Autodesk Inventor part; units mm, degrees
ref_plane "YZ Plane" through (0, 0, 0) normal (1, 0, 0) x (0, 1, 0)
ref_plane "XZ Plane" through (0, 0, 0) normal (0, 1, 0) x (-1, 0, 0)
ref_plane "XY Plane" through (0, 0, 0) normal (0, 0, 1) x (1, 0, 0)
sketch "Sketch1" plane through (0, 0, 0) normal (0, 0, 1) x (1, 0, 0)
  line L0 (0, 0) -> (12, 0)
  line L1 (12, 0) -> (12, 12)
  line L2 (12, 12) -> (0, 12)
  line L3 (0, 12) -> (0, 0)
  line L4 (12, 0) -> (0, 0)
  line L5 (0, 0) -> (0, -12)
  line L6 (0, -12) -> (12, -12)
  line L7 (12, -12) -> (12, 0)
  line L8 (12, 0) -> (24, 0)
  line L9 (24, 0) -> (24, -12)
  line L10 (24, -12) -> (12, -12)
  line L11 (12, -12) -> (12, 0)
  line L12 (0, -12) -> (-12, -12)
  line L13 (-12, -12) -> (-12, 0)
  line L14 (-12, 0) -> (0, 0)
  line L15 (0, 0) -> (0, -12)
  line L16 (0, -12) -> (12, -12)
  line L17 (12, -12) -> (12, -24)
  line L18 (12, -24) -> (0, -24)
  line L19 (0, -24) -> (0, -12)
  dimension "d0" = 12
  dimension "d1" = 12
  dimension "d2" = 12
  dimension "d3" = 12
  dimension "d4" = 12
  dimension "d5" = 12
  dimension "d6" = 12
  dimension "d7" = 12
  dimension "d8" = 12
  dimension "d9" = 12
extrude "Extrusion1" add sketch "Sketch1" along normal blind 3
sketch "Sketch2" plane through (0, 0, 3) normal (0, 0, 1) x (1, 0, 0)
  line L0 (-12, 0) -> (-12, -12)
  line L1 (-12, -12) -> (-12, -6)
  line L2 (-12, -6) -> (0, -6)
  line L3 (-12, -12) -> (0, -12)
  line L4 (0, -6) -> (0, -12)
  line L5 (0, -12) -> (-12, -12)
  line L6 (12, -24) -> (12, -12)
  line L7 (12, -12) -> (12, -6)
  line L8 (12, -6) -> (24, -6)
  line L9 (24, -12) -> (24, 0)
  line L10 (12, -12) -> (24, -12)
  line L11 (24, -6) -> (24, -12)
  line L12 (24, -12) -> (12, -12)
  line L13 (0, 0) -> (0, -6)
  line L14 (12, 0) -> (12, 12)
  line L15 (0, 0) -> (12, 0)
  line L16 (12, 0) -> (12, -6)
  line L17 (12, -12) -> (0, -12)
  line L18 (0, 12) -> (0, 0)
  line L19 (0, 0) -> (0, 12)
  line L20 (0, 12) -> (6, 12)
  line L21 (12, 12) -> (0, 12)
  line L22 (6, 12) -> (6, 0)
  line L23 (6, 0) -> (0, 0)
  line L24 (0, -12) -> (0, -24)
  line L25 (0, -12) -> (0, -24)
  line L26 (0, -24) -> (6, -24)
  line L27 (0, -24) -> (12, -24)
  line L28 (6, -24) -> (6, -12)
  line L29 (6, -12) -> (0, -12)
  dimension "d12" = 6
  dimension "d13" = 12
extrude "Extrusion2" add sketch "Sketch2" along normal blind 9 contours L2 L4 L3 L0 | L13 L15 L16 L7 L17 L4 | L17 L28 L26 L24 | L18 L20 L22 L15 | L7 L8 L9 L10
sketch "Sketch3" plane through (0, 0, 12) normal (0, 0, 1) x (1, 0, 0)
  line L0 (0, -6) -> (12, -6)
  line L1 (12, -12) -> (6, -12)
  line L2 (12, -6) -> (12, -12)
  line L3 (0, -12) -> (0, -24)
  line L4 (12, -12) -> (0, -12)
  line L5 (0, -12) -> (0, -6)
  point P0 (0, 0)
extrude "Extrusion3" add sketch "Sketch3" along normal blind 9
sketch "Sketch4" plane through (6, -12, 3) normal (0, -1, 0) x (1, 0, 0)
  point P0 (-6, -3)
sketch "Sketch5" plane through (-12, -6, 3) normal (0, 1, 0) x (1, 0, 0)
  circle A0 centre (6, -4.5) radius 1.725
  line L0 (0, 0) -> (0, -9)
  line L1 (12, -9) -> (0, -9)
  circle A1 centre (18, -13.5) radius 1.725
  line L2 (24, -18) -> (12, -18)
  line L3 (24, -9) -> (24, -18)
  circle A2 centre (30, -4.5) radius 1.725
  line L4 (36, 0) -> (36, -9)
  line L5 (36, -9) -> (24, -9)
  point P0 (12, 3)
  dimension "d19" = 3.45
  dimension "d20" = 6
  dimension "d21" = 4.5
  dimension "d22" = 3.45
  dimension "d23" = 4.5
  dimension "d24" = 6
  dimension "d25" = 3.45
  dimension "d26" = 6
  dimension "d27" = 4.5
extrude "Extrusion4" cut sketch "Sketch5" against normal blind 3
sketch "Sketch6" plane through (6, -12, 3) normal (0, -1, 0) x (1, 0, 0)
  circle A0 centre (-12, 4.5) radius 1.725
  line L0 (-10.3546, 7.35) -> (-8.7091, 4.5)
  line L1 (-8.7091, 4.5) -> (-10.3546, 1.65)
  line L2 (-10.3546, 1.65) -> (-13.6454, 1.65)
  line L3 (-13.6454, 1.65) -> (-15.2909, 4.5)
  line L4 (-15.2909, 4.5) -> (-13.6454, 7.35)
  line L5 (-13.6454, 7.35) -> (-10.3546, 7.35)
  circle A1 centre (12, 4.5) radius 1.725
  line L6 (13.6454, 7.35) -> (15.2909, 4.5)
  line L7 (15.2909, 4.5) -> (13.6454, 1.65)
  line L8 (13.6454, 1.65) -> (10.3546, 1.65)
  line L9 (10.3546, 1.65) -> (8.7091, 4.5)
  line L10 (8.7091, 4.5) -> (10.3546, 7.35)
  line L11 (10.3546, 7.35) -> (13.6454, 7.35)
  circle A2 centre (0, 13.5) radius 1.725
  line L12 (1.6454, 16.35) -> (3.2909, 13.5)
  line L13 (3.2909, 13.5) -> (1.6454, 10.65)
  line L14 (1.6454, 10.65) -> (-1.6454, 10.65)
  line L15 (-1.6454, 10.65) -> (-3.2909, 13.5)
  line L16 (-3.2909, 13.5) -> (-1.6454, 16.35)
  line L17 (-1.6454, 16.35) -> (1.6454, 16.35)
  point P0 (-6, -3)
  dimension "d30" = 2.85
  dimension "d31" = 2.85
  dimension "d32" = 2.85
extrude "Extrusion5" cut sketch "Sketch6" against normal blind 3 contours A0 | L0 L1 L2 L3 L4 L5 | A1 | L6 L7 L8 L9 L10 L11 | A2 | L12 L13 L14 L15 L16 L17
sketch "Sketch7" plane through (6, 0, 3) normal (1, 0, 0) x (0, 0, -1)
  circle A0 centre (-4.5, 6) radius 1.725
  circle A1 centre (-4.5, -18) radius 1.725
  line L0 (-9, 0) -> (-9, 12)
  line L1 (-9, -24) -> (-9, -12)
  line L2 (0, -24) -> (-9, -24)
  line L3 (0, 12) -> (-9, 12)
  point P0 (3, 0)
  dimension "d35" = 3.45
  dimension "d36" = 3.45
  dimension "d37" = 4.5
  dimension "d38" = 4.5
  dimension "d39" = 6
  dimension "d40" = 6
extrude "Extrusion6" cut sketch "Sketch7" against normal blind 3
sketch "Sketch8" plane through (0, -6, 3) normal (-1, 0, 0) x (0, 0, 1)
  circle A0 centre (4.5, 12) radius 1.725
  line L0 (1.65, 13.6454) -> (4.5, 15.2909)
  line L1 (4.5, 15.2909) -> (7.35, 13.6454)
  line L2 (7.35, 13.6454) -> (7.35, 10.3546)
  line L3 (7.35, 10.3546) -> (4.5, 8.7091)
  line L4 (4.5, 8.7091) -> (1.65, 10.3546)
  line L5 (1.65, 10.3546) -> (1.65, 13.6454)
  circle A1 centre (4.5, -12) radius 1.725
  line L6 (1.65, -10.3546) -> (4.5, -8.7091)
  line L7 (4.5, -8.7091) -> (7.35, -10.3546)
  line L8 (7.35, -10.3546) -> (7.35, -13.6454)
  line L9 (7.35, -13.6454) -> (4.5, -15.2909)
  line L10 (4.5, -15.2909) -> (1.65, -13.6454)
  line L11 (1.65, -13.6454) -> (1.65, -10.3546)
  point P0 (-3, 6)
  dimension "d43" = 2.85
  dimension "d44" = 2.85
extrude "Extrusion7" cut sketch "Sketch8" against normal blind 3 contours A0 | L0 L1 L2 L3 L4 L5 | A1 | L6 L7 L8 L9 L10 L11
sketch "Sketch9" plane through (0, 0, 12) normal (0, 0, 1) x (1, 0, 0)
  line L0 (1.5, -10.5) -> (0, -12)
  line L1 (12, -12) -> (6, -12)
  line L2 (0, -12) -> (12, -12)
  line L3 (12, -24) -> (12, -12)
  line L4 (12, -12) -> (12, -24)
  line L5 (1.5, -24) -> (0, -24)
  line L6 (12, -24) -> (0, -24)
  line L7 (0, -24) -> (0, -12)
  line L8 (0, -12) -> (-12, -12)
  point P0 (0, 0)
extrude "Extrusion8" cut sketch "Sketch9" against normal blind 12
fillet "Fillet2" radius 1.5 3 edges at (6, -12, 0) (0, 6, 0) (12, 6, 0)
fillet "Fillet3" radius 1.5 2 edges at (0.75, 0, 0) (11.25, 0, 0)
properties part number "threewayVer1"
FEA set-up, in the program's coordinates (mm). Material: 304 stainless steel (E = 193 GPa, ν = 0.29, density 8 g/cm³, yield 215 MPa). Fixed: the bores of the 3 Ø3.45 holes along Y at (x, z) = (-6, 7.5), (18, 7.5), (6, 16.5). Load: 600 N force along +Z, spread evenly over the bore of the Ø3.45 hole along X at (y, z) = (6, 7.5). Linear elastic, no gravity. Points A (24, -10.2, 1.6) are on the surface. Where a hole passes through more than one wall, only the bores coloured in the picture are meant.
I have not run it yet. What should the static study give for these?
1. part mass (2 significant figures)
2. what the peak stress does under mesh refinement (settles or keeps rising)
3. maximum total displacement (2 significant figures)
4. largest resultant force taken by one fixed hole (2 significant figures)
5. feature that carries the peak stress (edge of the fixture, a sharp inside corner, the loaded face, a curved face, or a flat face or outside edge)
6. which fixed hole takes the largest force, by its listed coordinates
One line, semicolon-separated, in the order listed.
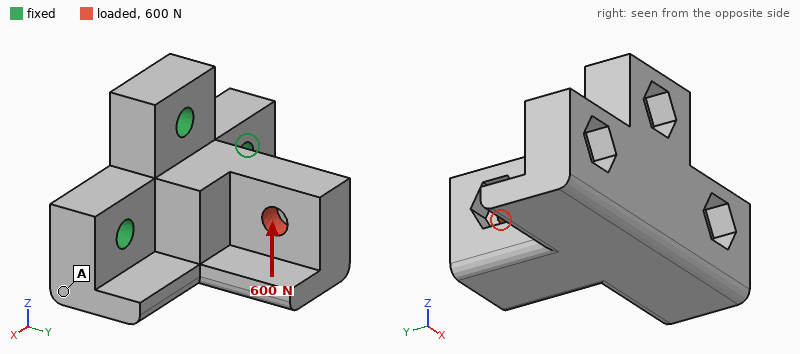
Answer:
41 g; keeps rising; 14 µm; 670 N; edge of the fixture; (6, 16.5)
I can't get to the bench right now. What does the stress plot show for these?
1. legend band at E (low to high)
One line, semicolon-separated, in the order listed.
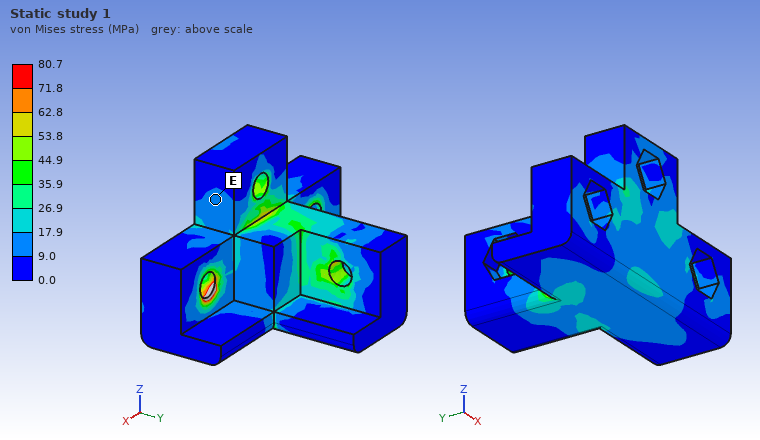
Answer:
9.0 to 17.9 MPa
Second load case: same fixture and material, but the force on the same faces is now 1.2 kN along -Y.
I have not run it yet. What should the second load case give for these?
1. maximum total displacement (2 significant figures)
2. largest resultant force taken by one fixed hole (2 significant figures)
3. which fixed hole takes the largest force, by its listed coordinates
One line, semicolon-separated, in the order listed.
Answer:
4.3 µm; 530 N; (-6, 7.5)
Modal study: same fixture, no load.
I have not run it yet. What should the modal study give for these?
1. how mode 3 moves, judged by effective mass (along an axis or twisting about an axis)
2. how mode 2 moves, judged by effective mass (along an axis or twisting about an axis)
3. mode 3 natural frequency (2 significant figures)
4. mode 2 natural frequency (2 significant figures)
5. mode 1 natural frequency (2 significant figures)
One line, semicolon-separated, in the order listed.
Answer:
along Y; along X; 26 kHz; 18 kHz; 12 kHz
